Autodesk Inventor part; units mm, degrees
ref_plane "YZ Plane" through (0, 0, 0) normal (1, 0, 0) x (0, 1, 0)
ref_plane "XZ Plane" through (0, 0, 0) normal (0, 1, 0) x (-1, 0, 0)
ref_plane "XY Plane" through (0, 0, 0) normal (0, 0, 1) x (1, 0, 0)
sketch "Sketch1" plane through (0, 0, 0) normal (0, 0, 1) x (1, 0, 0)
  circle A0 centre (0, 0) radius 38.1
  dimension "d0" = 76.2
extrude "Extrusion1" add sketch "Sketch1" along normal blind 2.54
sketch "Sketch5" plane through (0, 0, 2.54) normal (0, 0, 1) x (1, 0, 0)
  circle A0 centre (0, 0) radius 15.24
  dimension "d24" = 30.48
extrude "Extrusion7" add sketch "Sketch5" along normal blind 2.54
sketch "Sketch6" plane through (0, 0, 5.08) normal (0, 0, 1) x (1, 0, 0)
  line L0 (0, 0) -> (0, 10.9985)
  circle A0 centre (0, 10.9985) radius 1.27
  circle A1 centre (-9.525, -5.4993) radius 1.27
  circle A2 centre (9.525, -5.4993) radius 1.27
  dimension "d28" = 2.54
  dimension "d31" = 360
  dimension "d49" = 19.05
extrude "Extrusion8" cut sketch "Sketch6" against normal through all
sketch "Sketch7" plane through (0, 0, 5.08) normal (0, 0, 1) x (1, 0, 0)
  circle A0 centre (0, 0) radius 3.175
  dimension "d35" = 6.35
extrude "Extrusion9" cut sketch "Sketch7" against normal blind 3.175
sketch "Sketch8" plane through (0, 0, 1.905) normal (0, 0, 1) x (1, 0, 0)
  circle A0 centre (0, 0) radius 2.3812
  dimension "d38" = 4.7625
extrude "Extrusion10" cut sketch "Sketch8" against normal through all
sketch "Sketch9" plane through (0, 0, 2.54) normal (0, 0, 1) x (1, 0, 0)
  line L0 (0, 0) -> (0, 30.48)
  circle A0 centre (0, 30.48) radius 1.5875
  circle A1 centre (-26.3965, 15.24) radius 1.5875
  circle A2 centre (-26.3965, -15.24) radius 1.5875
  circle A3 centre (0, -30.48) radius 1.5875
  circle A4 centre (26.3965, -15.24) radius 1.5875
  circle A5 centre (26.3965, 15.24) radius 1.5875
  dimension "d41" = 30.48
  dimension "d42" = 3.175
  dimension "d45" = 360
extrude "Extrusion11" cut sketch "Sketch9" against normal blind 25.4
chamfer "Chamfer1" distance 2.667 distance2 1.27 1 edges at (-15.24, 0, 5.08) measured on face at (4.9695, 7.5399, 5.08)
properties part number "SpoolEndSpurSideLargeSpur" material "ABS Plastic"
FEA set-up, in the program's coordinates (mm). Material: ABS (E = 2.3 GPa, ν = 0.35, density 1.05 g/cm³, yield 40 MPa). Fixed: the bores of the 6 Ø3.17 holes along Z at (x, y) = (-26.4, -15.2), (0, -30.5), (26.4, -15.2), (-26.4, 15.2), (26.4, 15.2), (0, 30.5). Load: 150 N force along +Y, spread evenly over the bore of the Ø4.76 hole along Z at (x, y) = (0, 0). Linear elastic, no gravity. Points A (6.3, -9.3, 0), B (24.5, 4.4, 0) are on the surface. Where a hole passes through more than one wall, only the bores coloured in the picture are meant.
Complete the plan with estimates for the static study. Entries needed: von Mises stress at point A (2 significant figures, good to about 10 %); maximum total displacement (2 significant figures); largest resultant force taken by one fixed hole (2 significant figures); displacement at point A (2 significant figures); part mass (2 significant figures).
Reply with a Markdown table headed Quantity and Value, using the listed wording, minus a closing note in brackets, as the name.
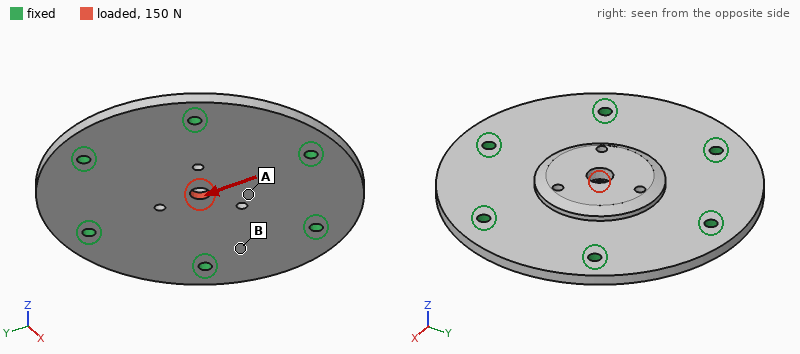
| Quantity | Value |
|---|---|
| von Mises stress at point A | 1.2 MPa |
| maximum total displacement | 22 µm |
| largest resultant force taken by one fixed hole | 37 N |
| displacement at point A | 11 µm |
| part mass | 14 g |
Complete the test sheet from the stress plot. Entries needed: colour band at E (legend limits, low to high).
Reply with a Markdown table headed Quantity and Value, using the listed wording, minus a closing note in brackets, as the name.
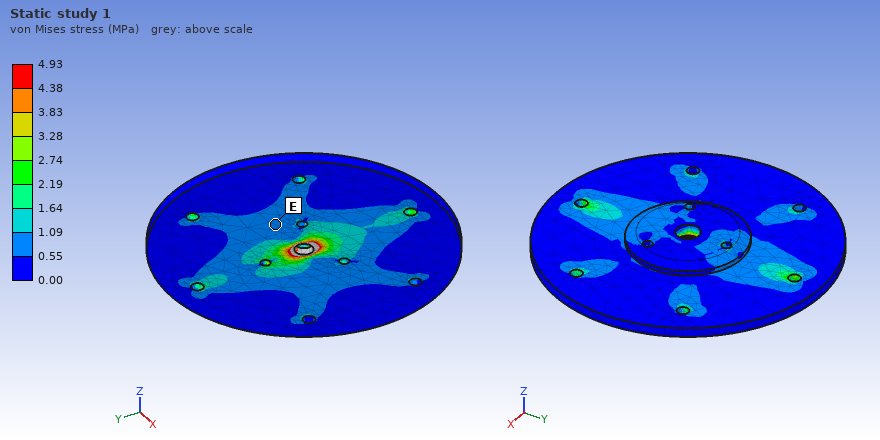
| Quantity | Value |
|---|---|
| colour band at E | 0.55 to 1.09 MPa |
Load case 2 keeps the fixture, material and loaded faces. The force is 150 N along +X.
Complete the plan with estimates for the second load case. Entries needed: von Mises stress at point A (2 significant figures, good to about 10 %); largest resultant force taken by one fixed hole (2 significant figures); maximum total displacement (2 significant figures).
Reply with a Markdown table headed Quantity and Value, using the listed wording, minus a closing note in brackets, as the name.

| Quantity | Value |
|---|---|
| von Mises stress at point A | 1.0 MPa |
| largest resultant force taken by one fixed hole | 33 N |
| maximum total displacement | 22 µm |
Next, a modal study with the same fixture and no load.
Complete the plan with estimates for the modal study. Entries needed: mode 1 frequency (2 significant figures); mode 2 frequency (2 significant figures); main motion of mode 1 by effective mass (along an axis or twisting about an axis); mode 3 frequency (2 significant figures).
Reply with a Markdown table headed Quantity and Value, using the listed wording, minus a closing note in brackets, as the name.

| Quantity | Value |
|---|---|
| mode 1 frequency | 1900 Hz |
| mode 2 frequency | 3100 Hz |
| main motion of mode 1 by effective mass | along Z |
| mode 3 frequency | 3200 Hz |
